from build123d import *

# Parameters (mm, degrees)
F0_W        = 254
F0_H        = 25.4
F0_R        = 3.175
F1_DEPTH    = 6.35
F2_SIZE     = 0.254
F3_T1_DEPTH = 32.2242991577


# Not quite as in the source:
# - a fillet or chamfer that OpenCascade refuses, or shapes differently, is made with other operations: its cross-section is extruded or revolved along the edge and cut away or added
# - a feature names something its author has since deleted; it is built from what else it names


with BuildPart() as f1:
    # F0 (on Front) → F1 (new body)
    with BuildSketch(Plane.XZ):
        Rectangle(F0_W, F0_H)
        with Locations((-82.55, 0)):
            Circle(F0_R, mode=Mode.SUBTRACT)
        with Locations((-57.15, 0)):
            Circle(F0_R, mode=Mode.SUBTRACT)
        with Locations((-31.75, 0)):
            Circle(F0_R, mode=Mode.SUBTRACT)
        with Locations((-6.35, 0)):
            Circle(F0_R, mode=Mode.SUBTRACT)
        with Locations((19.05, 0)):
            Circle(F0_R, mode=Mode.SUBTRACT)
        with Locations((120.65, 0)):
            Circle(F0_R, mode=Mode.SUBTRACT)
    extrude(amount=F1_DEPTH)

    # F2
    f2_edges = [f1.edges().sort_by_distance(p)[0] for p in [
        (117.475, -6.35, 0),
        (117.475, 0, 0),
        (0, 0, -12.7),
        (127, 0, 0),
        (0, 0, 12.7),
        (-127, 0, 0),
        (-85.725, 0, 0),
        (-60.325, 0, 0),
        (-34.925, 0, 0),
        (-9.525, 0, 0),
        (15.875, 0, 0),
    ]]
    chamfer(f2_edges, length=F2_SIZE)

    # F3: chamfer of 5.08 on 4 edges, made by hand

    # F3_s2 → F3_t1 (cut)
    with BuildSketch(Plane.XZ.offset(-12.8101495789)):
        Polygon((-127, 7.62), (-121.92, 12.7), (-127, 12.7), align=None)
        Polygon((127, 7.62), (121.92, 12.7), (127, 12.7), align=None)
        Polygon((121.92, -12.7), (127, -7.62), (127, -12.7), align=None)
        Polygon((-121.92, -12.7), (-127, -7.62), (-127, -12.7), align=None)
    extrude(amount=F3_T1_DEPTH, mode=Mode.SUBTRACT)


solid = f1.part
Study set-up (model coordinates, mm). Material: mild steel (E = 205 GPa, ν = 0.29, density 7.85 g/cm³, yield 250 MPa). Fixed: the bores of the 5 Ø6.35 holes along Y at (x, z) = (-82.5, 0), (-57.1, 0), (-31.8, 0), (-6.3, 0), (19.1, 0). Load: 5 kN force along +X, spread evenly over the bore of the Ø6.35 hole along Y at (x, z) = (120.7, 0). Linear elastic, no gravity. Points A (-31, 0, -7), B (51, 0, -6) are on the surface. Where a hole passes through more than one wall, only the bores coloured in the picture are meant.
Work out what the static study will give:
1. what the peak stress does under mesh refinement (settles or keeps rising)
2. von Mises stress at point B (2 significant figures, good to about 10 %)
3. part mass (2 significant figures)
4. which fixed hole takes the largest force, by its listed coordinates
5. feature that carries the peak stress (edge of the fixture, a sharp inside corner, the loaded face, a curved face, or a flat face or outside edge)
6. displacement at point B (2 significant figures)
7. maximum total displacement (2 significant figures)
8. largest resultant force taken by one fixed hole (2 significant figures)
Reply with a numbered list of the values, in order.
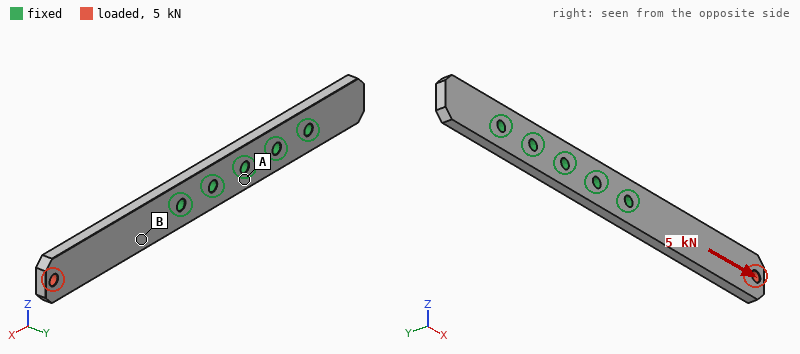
1. keeps rising
2. 31 MPa
3. 310 g
4. (19.1, 0)
5. edge of the fixture
6. 5.3 µm
7. 19 µm
8. 4.3 kN
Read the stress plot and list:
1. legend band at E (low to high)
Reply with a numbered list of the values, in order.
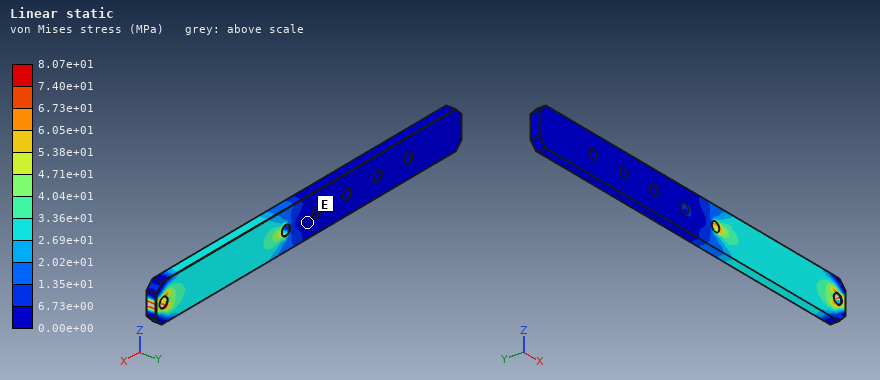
1. 0.00e+00 to 6.73e+00 MPa
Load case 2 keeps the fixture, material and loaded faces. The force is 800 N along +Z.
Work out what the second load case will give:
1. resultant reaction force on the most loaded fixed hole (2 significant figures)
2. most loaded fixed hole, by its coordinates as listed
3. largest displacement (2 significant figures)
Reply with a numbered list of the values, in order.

1. 2.7 kN
2. (19.1, 0)
3. 0.23 mm
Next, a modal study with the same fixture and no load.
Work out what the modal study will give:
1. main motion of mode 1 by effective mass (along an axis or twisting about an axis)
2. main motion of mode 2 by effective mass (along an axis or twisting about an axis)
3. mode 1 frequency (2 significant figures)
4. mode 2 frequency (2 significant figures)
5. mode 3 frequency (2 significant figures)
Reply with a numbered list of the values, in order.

1. along Y
2. along Z
3. 470 Hz
4. 1600 Hz
5. 2800 Hz
